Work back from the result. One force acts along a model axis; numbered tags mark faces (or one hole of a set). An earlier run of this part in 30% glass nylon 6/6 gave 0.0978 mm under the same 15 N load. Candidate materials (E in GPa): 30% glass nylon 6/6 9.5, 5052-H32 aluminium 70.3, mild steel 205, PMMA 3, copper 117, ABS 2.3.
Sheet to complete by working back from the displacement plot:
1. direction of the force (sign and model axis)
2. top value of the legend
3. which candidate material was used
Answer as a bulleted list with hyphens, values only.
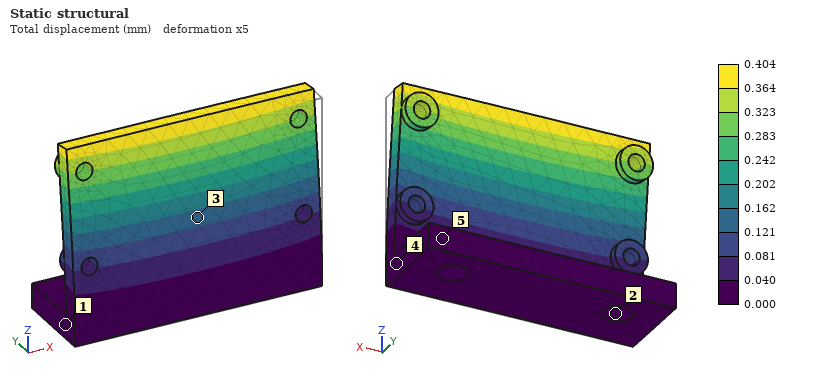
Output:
- +Y
- 0.404 mm
- ABS
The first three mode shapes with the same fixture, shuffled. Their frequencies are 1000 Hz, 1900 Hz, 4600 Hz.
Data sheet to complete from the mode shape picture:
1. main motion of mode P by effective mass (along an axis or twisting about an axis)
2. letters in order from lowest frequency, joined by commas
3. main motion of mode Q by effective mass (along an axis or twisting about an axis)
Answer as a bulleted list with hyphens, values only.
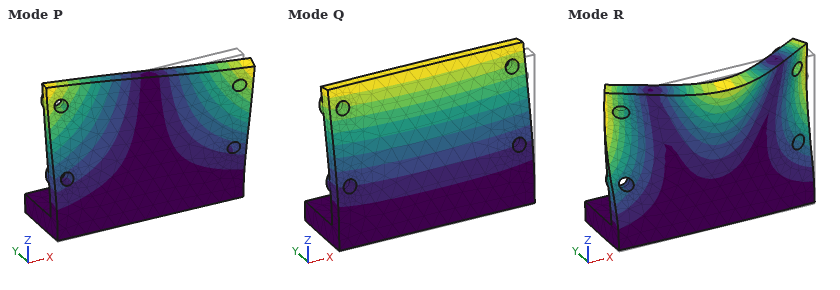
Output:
- twisting about Z
- Q, P, R
- along Y
